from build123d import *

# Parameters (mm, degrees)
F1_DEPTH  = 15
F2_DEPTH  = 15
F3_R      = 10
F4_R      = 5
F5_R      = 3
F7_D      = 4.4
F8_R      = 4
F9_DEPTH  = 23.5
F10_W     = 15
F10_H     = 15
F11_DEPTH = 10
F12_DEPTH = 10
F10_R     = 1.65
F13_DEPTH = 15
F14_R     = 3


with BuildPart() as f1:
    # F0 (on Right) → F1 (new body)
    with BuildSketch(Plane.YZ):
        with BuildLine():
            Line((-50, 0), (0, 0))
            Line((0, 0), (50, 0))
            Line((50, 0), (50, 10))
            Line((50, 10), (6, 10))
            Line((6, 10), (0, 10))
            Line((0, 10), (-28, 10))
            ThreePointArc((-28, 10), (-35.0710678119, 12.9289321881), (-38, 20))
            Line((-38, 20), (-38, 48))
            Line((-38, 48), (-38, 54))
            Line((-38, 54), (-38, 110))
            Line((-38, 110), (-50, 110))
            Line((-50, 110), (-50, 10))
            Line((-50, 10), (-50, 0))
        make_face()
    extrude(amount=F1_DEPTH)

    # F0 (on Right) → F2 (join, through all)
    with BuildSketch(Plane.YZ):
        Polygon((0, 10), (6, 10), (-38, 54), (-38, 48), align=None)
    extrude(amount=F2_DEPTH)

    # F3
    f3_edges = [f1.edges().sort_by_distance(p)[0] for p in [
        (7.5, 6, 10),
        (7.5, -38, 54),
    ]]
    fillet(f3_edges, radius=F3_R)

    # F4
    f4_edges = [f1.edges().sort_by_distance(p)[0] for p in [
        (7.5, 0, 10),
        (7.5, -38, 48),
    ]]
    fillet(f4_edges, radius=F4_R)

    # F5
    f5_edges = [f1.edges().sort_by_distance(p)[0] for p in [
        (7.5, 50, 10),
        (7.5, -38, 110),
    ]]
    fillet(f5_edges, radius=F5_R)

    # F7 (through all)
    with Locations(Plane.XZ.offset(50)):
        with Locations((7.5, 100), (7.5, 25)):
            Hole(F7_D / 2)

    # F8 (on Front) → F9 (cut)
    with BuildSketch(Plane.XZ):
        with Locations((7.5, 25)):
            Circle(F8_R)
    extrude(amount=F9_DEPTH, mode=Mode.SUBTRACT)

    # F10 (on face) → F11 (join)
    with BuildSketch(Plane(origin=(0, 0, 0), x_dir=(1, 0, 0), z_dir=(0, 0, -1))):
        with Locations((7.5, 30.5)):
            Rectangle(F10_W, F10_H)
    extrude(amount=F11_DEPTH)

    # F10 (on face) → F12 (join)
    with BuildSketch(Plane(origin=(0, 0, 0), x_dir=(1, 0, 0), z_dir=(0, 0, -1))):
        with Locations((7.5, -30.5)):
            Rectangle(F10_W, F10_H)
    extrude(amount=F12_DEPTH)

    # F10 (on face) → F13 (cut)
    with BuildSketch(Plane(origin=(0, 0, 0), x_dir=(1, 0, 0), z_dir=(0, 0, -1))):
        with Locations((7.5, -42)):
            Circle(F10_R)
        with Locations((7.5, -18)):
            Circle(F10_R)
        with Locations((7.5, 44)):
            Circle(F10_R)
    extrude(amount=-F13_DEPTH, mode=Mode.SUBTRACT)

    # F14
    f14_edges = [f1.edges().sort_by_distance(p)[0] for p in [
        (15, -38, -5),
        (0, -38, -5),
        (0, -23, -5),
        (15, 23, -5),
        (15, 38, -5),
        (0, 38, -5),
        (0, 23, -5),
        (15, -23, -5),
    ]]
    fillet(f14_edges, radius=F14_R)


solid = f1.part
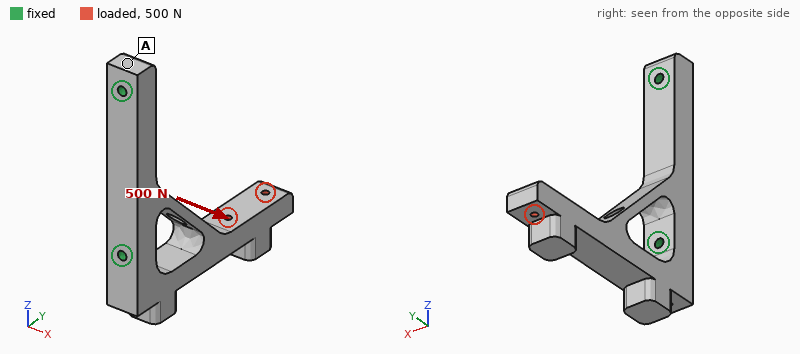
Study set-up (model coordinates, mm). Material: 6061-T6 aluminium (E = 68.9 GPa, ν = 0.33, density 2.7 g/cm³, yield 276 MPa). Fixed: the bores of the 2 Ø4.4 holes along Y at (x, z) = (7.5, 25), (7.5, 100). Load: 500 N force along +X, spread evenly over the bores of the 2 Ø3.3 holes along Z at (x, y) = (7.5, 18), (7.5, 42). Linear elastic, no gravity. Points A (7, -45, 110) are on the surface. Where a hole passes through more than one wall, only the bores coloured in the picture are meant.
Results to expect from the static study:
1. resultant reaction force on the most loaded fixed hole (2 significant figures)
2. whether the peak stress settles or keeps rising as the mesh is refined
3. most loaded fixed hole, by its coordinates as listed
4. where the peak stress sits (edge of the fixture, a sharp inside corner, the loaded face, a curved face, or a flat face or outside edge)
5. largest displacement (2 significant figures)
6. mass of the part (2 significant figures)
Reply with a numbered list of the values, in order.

1. 610 N
2. keeps rising
3. (7.5, 25)
4. edge of the fixture
5. 0.61 mm
6. 110 g
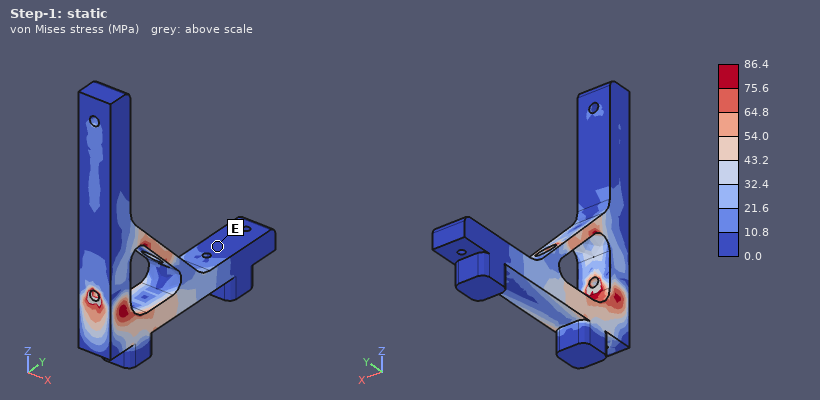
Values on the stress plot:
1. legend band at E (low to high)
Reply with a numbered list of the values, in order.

1. 0.0 to 10.8 MPa
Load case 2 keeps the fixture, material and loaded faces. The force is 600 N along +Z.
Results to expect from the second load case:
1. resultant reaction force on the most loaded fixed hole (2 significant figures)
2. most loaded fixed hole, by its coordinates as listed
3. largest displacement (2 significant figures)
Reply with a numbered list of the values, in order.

1. 510 N
2. (7.5, 100)
3. 0.28 mm
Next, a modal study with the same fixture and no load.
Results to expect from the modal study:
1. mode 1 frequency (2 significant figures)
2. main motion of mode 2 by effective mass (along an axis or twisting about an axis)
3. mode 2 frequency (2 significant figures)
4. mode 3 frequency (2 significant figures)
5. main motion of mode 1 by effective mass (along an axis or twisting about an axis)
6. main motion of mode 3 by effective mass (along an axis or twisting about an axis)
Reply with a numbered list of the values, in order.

1. 1000 Hz
2. along Z
3. 1800 Hz
4. 4200 Hz
5. along X
6. along Y
